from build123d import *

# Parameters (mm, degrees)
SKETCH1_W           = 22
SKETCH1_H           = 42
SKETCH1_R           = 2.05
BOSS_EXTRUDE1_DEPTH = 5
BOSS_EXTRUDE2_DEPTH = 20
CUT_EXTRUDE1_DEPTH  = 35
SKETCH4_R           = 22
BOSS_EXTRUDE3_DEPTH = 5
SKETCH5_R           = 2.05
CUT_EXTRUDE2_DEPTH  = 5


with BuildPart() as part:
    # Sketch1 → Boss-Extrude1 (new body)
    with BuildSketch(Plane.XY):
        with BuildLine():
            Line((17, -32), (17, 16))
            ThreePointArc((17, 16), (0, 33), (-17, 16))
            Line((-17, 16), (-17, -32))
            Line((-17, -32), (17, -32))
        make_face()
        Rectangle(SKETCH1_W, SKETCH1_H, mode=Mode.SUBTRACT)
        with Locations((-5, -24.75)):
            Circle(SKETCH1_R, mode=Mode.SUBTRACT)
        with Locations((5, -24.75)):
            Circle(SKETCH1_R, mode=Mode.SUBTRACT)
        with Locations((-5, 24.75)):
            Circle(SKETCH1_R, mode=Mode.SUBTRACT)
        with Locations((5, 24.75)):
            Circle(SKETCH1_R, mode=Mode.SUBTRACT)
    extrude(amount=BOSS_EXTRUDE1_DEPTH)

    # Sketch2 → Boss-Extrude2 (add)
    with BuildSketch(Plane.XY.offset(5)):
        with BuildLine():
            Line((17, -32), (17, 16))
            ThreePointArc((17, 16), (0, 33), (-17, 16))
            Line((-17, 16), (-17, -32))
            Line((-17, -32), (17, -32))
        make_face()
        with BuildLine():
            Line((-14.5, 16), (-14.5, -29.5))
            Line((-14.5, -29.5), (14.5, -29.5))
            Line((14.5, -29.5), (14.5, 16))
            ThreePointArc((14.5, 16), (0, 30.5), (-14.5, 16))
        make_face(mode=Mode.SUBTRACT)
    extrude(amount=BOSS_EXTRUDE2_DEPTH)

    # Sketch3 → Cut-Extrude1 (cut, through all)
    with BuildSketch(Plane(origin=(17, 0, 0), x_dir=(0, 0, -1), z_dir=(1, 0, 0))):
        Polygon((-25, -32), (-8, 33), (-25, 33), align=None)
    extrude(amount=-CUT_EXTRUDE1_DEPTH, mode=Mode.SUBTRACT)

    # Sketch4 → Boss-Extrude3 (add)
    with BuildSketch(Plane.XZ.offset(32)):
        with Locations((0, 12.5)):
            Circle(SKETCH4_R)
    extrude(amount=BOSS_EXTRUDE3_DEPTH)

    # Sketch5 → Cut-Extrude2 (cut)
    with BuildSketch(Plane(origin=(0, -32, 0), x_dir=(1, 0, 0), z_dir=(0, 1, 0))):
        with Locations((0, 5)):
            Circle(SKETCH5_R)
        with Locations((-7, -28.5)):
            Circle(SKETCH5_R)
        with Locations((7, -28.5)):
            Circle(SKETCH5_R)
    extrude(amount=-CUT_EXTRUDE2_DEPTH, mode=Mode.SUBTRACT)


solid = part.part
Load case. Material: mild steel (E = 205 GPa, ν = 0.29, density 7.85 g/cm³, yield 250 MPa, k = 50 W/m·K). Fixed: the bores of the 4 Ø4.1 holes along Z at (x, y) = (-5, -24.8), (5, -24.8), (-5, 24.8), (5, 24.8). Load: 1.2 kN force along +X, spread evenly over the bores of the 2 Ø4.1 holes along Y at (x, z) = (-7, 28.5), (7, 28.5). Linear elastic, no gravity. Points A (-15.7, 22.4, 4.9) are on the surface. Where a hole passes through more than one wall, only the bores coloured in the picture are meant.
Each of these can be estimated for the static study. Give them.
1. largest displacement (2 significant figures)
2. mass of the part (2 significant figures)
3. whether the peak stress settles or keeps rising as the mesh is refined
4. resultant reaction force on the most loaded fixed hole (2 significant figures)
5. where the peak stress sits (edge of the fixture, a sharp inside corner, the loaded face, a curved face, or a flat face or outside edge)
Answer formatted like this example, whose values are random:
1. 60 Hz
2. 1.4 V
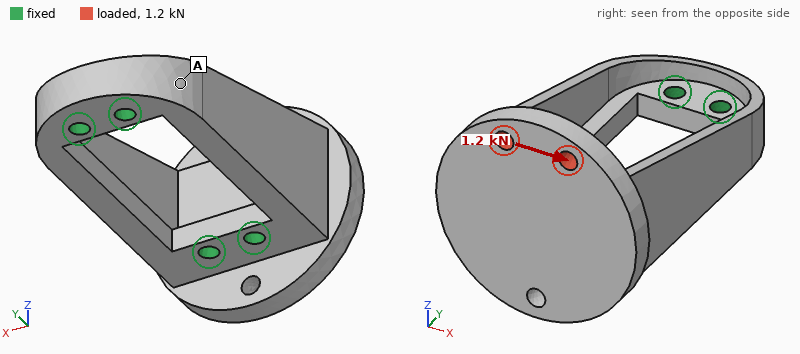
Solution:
1. 26 µm
2. 140 g
3. keeps rising
4. 2.0 kN
5. edge of the fixture
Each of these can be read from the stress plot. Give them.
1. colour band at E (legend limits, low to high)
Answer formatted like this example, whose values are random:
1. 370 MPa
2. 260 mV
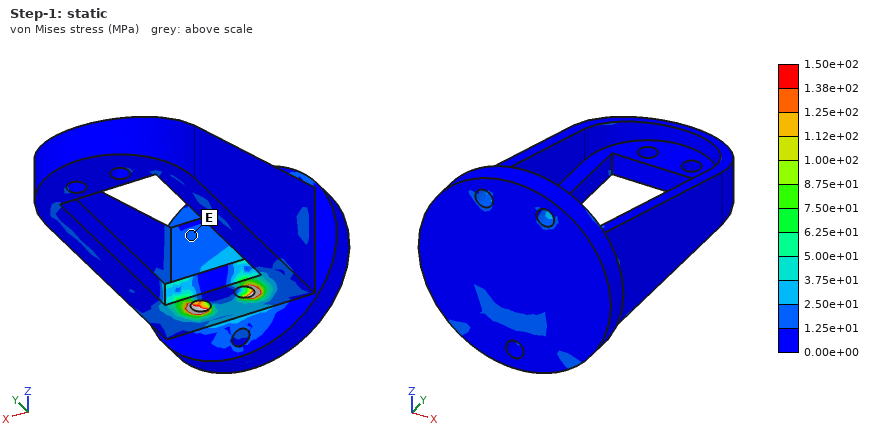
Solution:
1. 1.25e+01 to 2.50e+01 MPa
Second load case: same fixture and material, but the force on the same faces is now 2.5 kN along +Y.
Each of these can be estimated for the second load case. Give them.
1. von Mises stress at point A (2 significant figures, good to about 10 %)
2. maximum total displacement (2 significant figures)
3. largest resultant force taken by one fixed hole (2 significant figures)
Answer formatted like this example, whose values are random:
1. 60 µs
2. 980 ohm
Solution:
1. 51 MPa
2. 70 µm
3. 870 N
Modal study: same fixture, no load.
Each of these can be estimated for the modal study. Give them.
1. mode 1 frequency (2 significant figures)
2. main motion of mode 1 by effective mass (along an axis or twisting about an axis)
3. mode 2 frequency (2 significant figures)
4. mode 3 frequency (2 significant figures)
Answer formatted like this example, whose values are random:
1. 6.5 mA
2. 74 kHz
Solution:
1. 5800 Hz
2. along X
3. 6400 Hz
4. 7700 Hz
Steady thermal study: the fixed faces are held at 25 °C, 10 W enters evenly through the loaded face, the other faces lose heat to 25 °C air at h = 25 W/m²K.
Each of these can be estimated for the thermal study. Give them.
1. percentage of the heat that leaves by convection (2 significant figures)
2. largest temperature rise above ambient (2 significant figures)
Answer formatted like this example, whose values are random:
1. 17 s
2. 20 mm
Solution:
1. 18 %
2. 29 K
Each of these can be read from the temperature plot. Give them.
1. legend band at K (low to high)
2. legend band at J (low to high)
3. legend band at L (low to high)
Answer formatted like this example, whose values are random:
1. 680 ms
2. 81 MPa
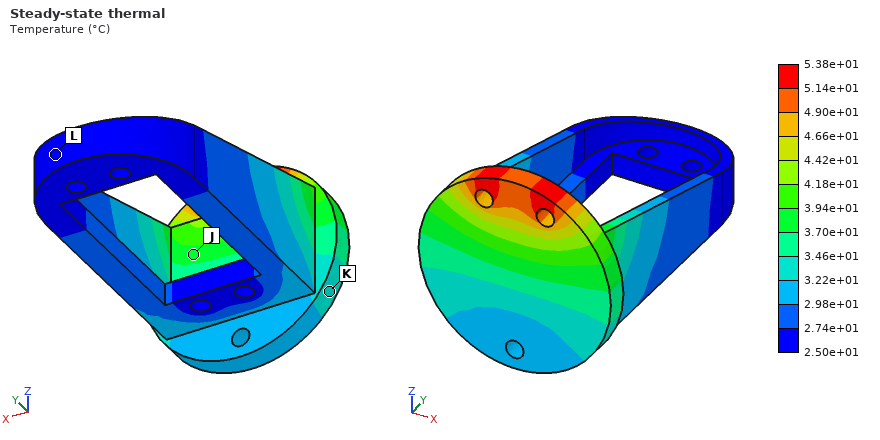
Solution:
1. 3.22e+01 to 3.46e+01 °C
2. 3.70e+01 to 3.94e+01 °C
3. 2.50e+01 to 2.74e+01 °C
